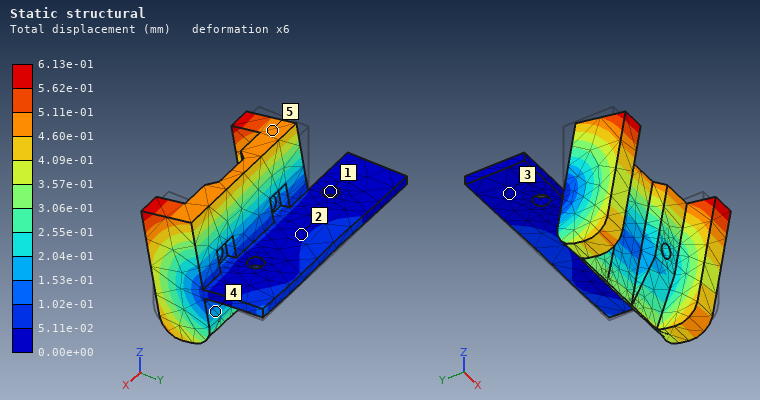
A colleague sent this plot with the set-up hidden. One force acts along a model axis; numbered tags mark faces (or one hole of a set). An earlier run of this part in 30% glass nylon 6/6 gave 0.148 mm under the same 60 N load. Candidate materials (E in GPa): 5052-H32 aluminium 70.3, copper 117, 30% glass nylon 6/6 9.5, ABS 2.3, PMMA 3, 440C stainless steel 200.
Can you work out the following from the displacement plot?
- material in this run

ABS
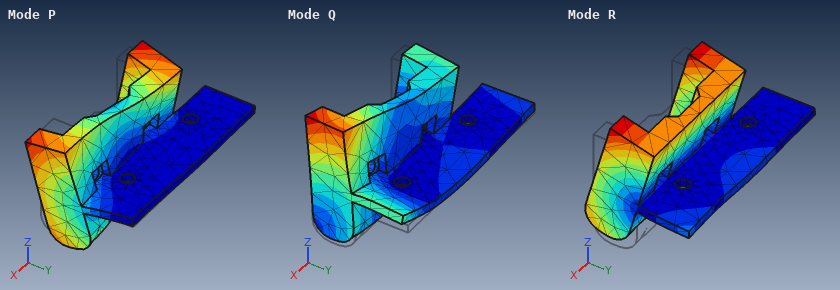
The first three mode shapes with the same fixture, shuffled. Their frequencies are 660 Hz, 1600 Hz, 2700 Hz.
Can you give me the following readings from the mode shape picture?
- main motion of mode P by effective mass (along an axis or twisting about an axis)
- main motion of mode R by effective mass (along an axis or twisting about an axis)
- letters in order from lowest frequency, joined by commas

twisting about Y
along Z
R, P, Q
